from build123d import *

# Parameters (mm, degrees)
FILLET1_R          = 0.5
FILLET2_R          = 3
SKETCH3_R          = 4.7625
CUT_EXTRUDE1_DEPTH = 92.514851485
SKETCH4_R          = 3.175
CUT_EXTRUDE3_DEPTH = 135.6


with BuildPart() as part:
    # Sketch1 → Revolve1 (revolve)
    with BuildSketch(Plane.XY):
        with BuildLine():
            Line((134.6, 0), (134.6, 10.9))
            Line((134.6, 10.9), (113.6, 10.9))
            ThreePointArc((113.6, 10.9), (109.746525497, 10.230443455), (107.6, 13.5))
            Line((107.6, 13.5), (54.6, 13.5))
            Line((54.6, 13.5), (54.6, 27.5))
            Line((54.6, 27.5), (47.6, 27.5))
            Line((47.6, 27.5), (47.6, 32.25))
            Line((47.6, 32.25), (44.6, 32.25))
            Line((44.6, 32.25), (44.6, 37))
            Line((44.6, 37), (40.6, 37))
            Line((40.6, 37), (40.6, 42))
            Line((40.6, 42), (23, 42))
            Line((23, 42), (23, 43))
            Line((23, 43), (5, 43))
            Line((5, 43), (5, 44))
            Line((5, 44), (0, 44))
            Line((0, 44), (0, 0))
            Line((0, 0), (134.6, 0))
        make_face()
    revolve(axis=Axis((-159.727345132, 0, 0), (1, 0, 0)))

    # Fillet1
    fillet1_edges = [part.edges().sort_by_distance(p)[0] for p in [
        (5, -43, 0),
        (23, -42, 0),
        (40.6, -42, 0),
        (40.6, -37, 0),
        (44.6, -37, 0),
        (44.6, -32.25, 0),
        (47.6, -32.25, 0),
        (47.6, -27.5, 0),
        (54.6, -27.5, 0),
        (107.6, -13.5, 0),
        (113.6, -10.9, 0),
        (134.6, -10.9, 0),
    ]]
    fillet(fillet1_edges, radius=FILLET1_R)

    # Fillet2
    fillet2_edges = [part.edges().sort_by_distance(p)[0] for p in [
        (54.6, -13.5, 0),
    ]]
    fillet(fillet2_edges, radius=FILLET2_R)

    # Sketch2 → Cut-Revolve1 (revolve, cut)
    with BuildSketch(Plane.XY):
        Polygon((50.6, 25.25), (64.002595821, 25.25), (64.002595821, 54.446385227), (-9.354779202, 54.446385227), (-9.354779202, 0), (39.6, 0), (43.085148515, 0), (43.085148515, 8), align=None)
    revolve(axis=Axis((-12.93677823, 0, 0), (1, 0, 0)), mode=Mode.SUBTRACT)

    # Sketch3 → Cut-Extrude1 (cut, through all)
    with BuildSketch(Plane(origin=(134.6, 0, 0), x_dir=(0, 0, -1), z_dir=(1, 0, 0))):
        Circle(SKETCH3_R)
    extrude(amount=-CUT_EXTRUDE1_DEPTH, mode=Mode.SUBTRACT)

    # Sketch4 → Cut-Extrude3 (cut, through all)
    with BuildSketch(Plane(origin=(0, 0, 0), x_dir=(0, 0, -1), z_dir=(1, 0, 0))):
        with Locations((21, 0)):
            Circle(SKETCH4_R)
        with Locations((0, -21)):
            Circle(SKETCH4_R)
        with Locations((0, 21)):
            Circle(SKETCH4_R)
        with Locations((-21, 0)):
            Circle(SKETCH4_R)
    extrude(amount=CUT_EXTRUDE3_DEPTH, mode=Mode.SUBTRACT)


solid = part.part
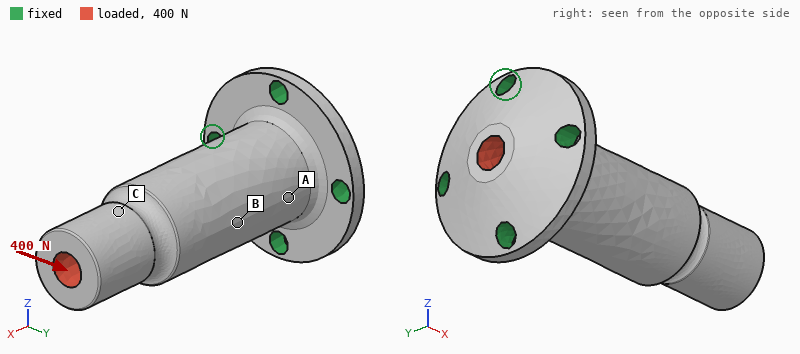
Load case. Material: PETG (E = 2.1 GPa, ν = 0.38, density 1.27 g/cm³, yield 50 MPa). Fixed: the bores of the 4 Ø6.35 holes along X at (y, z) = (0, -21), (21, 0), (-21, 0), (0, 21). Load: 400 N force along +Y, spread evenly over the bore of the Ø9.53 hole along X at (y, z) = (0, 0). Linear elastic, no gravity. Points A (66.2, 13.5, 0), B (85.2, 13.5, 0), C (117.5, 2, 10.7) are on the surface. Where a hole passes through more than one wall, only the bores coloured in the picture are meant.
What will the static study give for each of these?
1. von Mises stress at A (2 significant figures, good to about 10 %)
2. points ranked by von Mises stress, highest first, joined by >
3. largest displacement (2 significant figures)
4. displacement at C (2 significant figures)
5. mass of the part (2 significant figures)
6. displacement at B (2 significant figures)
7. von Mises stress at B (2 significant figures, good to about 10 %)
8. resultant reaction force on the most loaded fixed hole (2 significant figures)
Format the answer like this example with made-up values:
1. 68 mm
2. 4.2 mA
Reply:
1. 5.4 MPa
2. A > B > C
3. 0.70 mm
4. 0.52 mm
5. 61 g
6. 0.24 mm
7. 2.8 MPa
8. 420 N
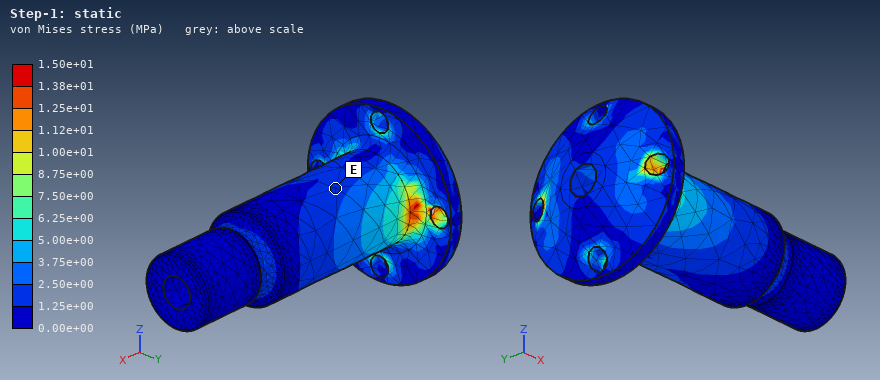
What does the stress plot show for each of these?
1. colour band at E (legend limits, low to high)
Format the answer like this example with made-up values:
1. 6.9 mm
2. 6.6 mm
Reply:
1. 1.25e+00 to 2.50e+00 MPa
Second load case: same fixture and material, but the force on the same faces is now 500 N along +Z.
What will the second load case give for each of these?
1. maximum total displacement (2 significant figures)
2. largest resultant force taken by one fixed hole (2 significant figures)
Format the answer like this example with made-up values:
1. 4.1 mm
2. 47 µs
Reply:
1. 0.88 mm
2. 520 N
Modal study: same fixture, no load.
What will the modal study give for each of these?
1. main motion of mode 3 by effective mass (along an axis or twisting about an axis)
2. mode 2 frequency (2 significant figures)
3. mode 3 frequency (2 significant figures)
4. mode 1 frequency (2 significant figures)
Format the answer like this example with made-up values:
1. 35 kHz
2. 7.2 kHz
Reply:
1. twisting about X
2. 740 Hz
3. 2800 Hz
4. 740 Hz
